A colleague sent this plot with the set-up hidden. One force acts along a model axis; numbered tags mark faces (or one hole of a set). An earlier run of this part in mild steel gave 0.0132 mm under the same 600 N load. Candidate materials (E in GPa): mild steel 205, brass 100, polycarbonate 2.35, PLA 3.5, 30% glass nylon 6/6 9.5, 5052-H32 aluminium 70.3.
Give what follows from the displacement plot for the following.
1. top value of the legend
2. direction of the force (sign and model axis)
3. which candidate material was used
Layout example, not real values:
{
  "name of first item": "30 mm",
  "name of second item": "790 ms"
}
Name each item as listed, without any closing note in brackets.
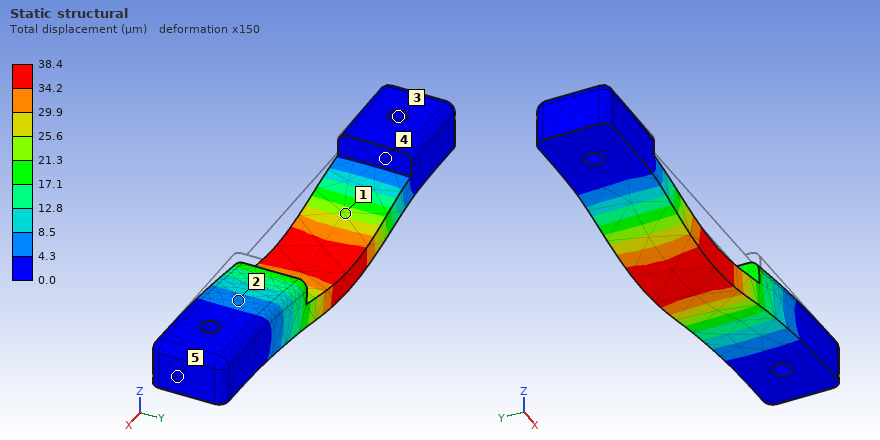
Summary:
{
  "top value of the legend": "38.4 µm",
  "direction of the force": "-Z",
  "which candidate material was used": "5052-H32 aluminium"
}
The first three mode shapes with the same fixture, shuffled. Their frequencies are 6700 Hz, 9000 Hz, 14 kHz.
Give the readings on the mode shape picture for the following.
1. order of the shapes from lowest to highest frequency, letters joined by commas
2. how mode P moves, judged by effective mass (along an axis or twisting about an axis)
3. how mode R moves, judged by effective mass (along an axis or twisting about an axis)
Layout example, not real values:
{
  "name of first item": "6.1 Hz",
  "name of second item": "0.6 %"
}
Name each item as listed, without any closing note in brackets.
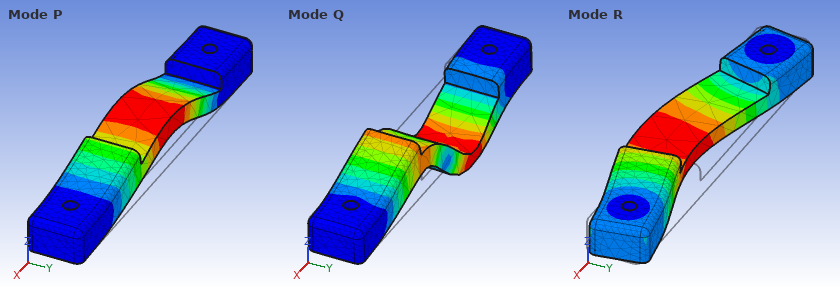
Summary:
{
  "order of the shapes from lowest to highest frequency, letters joined by commas": "P, R, Q",
  "how mode P moves, judged by effective mass": "along Z",
  "how mode R moves, judged by effective mass": "along Y"
}
